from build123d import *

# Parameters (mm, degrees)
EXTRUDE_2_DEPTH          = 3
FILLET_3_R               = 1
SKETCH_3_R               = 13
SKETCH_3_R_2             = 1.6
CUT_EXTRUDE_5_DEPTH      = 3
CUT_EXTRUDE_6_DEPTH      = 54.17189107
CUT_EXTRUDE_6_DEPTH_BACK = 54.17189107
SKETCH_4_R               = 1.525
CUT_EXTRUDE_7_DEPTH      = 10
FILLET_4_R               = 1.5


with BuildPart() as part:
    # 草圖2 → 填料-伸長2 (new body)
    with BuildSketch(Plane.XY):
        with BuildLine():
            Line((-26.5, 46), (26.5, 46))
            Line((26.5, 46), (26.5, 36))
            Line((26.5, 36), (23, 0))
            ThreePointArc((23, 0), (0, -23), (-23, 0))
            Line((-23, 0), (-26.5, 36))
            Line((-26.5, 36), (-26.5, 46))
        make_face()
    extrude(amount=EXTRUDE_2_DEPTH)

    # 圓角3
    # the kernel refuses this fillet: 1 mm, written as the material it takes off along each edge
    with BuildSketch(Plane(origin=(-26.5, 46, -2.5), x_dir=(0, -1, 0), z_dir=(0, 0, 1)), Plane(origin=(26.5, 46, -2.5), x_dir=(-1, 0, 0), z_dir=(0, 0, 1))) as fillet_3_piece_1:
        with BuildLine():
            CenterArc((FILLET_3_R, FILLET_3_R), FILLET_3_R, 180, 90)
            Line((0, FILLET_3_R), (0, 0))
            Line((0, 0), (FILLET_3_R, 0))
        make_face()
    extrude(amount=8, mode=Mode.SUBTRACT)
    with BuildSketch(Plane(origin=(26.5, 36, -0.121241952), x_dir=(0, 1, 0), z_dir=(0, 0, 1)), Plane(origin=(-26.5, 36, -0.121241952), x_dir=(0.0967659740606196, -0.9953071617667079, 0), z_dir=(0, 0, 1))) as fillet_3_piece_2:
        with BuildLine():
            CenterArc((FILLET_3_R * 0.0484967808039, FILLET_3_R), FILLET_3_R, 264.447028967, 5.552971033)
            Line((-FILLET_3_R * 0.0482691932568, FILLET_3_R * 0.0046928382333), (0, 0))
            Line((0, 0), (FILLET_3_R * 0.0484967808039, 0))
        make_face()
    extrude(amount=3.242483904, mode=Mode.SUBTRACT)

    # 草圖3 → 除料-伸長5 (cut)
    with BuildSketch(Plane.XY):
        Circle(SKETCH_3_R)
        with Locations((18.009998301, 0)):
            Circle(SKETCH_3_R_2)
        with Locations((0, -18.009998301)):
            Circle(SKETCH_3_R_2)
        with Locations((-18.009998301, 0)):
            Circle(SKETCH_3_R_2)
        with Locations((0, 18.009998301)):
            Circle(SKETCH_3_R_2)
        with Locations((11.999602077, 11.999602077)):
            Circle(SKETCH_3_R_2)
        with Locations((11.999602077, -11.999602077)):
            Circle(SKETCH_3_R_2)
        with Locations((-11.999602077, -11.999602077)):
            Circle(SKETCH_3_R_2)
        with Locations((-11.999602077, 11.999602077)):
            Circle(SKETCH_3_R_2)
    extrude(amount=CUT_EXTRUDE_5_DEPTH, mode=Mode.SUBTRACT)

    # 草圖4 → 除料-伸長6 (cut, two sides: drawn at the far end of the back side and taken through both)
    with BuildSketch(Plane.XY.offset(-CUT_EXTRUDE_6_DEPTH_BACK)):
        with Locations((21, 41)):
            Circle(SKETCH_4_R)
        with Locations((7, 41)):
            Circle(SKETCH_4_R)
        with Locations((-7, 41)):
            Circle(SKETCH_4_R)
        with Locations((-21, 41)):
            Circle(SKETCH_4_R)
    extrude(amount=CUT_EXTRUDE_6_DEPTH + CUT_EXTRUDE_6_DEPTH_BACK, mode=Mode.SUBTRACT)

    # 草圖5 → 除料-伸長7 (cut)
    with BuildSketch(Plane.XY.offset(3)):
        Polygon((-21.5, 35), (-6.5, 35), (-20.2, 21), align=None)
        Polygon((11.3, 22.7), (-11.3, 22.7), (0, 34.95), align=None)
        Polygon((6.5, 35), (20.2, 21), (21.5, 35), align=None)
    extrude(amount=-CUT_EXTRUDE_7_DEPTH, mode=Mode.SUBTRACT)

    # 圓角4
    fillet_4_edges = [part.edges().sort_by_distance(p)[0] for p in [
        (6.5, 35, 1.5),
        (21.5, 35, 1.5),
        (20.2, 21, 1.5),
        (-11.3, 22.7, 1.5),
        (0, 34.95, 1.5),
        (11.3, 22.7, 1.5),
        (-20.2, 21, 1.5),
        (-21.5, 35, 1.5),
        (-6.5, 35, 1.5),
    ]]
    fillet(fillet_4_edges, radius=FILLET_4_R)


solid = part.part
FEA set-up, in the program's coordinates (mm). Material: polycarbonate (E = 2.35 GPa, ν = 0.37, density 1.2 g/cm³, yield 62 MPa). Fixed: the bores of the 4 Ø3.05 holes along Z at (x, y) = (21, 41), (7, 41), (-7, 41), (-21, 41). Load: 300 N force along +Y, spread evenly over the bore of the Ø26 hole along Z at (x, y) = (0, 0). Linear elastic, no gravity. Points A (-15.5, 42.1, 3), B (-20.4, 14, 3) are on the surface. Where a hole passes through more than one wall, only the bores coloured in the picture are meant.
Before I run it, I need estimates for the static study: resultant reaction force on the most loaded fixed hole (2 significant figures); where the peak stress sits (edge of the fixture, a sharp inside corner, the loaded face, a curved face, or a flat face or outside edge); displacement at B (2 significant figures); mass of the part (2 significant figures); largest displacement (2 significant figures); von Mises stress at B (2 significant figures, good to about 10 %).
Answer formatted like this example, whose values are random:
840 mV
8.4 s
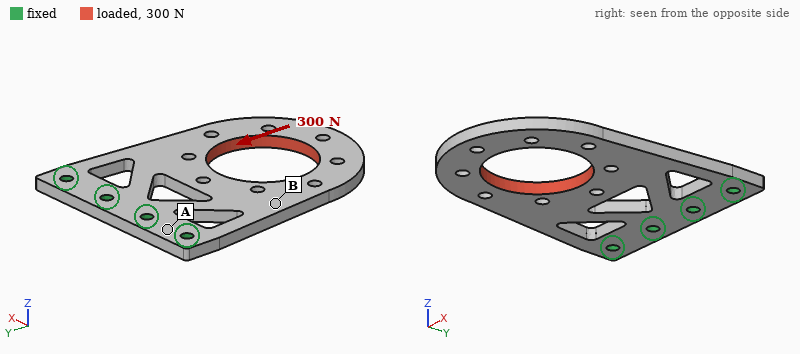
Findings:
85 N
a curved face
0.063 mm
7.9 g
0.13 mm
3.5 MPa
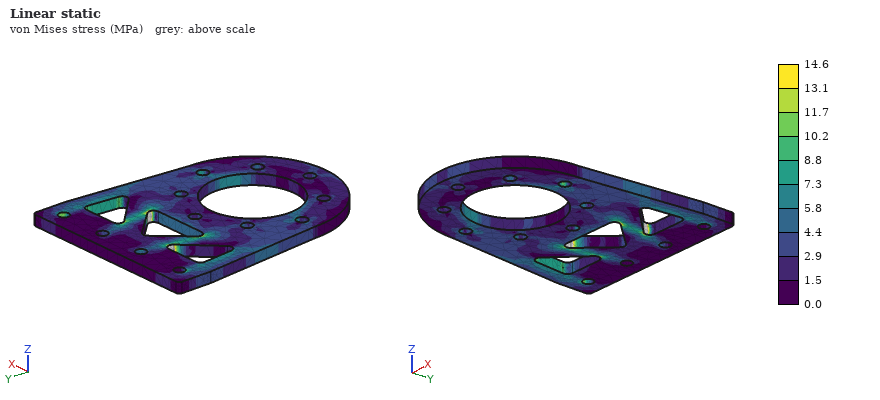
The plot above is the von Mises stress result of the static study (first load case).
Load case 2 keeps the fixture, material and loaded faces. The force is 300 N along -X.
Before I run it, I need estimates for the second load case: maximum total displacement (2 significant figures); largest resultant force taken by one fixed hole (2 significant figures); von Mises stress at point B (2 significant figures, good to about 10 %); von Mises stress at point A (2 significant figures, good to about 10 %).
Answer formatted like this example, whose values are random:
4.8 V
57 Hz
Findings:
0.84 mm
270 N
6.2 MPa
2.6 MPa
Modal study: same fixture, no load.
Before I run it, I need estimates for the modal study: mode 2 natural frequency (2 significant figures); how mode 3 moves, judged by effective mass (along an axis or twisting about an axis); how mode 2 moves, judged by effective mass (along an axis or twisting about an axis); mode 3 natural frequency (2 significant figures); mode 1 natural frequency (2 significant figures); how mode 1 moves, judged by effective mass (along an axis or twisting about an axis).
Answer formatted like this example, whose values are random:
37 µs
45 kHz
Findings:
530 Hz
along Z
twisting about Y
930 Hz
170 Hz
along Z
